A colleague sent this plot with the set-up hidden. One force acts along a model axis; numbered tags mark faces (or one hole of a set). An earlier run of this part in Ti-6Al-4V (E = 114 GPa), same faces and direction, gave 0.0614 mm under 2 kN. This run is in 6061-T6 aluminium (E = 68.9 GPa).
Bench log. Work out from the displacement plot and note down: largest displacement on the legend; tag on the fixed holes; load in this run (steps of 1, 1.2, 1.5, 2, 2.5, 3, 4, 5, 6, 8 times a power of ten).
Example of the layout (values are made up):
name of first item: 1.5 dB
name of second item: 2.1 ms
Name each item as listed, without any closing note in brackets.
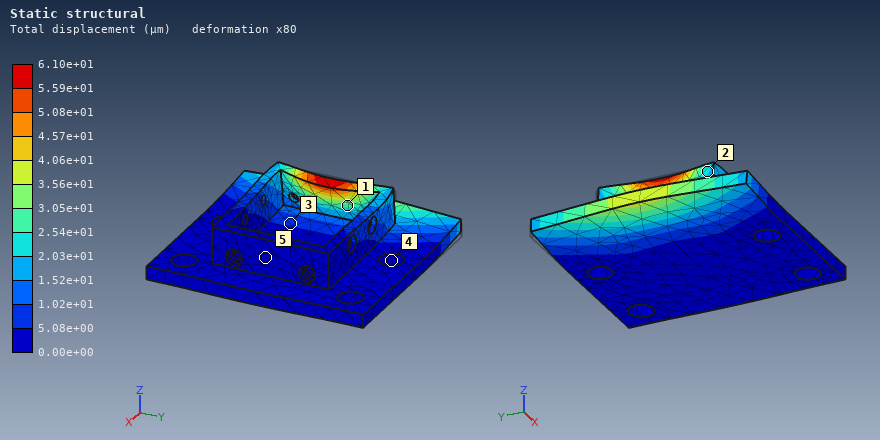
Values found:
largest displacement on the legend: 6.10e+01 µm
tag on the fixed holes: 4
load in this run: 1.2 kN
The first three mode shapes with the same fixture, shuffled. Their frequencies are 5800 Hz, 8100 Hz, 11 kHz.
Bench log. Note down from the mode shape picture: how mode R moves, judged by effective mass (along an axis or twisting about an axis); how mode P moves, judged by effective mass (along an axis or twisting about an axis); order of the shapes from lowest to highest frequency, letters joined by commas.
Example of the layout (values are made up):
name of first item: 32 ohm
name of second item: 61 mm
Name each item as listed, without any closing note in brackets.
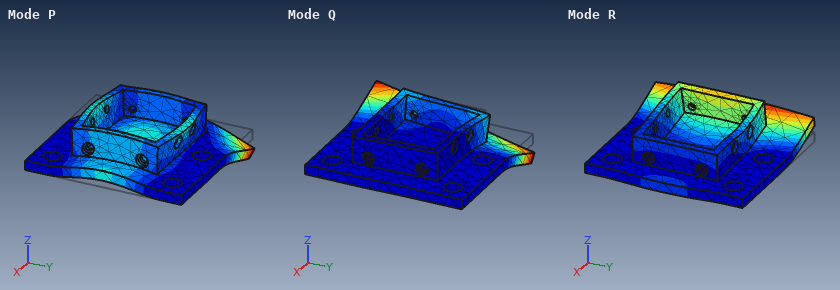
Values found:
how mode R moves, judged by effective mass: along Z
how mode P moves, judged by effective mass: along Z
order of the shapes from lowest to highest frequency, letters joined by commas: R, Q, P
